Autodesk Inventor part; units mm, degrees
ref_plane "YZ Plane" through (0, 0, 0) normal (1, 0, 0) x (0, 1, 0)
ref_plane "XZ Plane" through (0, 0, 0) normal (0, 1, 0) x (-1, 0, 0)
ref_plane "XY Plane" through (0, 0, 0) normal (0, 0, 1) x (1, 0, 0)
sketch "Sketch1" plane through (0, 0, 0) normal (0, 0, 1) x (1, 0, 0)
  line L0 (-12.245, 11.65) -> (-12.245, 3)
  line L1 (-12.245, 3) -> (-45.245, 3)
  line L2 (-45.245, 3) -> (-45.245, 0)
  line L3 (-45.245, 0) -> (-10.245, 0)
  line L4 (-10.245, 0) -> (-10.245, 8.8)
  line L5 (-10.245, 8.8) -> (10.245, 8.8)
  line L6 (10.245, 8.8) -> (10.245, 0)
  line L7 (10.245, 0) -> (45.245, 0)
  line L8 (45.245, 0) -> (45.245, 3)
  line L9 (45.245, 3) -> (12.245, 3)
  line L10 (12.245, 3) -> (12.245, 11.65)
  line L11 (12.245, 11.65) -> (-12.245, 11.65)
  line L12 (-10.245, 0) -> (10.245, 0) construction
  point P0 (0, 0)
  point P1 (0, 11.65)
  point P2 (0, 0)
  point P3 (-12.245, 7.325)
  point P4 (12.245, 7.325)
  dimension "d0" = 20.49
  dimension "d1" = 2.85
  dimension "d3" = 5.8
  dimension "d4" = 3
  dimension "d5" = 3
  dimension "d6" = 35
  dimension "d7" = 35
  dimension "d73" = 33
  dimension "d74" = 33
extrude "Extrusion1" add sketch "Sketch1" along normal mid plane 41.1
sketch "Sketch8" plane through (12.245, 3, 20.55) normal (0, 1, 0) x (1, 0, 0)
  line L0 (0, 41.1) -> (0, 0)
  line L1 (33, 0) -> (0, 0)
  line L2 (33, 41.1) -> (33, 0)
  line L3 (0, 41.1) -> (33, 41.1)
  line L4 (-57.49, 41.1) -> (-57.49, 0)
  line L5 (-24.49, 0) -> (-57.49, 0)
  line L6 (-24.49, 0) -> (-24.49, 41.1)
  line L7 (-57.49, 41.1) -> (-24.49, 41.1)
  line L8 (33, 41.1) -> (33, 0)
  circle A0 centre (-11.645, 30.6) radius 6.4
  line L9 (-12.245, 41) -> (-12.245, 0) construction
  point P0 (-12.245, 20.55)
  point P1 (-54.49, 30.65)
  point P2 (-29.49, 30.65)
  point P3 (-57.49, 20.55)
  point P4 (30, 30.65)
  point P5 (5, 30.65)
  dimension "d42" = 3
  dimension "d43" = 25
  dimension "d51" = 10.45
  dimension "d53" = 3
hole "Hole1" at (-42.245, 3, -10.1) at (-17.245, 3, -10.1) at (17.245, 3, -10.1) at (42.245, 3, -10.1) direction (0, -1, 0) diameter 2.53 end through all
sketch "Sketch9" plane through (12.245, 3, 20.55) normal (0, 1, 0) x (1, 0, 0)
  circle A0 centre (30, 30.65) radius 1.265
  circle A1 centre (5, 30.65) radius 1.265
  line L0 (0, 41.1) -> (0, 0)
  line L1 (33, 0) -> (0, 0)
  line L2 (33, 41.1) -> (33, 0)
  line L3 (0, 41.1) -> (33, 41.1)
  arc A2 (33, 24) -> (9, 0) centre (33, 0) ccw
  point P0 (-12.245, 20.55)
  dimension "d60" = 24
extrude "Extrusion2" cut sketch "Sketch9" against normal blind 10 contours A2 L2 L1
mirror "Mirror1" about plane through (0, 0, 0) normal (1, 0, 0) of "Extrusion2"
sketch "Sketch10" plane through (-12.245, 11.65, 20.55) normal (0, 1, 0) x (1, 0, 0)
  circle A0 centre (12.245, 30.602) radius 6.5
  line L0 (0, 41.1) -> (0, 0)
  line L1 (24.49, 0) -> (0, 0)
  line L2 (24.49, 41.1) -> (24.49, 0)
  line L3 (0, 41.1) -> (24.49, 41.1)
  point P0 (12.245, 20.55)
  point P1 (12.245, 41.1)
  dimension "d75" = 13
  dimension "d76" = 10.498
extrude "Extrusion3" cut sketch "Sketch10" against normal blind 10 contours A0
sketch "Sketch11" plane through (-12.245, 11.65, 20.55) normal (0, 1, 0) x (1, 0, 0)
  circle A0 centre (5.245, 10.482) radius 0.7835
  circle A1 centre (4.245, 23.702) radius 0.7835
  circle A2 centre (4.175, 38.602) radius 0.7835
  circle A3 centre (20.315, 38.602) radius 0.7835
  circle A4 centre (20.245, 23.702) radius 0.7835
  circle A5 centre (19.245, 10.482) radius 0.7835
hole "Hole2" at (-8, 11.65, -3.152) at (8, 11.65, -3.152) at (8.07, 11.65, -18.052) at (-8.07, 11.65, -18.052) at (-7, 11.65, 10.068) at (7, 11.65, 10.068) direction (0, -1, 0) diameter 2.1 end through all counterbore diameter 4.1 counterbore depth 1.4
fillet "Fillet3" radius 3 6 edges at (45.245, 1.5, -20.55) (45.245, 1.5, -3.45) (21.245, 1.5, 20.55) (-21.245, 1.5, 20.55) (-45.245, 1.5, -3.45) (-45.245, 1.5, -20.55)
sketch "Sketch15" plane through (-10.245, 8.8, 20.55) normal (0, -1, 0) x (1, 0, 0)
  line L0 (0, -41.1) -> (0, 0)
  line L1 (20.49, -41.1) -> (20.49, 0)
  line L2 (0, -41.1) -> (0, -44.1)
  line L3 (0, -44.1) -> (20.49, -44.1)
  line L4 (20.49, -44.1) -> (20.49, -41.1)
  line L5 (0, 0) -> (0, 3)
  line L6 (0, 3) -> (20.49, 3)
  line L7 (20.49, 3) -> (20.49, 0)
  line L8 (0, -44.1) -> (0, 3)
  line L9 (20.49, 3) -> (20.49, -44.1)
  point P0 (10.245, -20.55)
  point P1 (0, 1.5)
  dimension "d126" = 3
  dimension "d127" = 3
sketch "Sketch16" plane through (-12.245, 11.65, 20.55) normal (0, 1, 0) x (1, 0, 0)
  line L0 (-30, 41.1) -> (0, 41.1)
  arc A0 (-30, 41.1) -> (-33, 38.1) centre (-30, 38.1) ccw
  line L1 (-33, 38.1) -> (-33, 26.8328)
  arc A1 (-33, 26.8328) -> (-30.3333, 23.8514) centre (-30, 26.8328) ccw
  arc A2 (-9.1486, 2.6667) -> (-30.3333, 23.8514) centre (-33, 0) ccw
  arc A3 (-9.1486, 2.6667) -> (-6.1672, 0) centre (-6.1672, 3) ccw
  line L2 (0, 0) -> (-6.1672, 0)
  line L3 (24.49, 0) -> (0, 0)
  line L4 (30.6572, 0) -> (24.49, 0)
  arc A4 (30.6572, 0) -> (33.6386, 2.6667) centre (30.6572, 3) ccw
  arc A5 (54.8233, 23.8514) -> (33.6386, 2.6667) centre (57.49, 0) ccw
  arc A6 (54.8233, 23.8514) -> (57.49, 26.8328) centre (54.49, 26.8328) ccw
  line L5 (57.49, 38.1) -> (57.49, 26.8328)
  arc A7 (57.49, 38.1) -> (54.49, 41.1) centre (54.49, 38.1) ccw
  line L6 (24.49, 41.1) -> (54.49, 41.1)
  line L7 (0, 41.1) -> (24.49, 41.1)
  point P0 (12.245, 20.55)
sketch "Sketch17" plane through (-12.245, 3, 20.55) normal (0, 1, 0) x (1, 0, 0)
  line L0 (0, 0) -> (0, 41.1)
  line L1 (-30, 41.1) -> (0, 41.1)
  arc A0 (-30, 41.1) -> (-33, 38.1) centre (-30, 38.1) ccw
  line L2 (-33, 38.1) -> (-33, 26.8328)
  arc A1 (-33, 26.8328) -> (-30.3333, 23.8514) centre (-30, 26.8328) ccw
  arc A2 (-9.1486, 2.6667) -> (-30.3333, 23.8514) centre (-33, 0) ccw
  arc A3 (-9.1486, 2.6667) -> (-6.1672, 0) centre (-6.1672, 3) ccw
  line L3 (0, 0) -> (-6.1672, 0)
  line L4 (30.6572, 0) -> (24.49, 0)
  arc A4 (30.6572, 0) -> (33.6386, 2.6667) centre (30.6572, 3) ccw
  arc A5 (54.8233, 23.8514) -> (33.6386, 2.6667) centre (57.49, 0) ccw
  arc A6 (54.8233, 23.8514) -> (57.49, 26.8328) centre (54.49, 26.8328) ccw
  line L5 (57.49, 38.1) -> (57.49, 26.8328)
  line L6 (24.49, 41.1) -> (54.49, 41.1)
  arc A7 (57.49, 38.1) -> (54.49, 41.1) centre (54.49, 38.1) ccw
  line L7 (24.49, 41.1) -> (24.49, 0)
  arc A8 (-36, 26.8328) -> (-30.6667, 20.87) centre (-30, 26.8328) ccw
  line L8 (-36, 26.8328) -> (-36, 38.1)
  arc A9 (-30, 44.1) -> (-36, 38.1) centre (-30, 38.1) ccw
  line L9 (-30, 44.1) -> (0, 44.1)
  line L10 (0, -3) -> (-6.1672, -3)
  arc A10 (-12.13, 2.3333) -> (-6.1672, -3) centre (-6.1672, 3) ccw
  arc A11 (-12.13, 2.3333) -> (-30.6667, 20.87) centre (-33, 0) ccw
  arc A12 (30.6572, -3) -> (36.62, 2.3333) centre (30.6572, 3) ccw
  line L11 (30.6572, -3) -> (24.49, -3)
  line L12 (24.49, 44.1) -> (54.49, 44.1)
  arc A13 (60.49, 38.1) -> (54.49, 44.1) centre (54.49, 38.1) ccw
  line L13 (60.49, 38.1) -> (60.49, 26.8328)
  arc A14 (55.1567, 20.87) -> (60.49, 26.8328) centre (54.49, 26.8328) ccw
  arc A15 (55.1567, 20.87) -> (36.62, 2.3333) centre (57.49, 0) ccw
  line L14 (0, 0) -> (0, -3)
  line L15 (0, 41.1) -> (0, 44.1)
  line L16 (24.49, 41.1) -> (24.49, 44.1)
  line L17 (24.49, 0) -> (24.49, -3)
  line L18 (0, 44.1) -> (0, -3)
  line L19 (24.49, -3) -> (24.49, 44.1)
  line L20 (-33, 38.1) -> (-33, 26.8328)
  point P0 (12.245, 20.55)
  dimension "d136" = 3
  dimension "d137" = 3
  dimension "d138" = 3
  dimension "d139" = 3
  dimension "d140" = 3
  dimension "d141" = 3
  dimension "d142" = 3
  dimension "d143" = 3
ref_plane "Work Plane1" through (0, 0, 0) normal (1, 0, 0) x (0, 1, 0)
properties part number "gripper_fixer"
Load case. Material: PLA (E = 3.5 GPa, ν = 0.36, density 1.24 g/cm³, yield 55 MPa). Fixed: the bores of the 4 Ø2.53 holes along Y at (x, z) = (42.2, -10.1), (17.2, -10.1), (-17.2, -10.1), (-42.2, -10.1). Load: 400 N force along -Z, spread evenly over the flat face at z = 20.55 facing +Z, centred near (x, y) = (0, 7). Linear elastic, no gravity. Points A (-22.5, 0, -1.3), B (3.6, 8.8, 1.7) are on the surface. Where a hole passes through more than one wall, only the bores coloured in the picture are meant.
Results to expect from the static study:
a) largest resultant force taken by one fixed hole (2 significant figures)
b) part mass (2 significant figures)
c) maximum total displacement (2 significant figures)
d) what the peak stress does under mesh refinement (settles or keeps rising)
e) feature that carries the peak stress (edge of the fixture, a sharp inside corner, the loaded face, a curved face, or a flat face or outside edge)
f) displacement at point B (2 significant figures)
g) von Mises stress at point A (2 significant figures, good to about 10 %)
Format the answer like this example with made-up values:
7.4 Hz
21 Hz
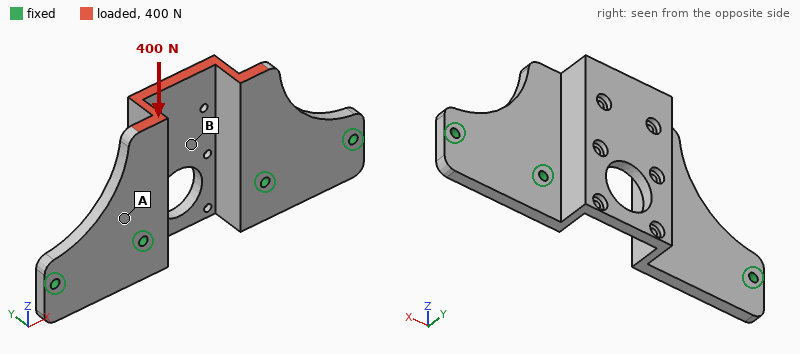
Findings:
240 N
11 g
0.85 mm
keeps rising
edge of the fixture
0.37 mm
7.7 MPa
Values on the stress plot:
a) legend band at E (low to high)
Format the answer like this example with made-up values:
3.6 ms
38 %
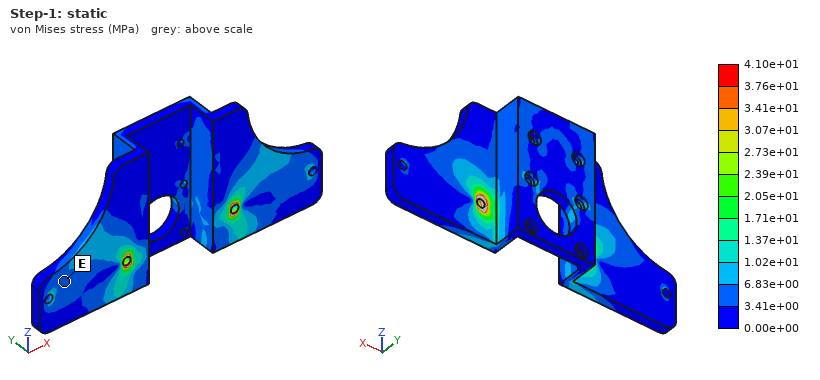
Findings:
3.41e+00 to 6.83e+00 MPa
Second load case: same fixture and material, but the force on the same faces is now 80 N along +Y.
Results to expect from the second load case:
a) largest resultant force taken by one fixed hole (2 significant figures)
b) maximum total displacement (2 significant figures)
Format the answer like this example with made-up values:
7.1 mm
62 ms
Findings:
51 N
1.1 mm
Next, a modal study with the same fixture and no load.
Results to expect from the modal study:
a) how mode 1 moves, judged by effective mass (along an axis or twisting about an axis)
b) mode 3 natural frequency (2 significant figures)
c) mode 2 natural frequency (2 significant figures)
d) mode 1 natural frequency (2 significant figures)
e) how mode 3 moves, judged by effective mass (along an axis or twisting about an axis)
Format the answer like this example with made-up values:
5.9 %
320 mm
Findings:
along Y
3200 Hz
2200 Hz
970 Hz
along X
